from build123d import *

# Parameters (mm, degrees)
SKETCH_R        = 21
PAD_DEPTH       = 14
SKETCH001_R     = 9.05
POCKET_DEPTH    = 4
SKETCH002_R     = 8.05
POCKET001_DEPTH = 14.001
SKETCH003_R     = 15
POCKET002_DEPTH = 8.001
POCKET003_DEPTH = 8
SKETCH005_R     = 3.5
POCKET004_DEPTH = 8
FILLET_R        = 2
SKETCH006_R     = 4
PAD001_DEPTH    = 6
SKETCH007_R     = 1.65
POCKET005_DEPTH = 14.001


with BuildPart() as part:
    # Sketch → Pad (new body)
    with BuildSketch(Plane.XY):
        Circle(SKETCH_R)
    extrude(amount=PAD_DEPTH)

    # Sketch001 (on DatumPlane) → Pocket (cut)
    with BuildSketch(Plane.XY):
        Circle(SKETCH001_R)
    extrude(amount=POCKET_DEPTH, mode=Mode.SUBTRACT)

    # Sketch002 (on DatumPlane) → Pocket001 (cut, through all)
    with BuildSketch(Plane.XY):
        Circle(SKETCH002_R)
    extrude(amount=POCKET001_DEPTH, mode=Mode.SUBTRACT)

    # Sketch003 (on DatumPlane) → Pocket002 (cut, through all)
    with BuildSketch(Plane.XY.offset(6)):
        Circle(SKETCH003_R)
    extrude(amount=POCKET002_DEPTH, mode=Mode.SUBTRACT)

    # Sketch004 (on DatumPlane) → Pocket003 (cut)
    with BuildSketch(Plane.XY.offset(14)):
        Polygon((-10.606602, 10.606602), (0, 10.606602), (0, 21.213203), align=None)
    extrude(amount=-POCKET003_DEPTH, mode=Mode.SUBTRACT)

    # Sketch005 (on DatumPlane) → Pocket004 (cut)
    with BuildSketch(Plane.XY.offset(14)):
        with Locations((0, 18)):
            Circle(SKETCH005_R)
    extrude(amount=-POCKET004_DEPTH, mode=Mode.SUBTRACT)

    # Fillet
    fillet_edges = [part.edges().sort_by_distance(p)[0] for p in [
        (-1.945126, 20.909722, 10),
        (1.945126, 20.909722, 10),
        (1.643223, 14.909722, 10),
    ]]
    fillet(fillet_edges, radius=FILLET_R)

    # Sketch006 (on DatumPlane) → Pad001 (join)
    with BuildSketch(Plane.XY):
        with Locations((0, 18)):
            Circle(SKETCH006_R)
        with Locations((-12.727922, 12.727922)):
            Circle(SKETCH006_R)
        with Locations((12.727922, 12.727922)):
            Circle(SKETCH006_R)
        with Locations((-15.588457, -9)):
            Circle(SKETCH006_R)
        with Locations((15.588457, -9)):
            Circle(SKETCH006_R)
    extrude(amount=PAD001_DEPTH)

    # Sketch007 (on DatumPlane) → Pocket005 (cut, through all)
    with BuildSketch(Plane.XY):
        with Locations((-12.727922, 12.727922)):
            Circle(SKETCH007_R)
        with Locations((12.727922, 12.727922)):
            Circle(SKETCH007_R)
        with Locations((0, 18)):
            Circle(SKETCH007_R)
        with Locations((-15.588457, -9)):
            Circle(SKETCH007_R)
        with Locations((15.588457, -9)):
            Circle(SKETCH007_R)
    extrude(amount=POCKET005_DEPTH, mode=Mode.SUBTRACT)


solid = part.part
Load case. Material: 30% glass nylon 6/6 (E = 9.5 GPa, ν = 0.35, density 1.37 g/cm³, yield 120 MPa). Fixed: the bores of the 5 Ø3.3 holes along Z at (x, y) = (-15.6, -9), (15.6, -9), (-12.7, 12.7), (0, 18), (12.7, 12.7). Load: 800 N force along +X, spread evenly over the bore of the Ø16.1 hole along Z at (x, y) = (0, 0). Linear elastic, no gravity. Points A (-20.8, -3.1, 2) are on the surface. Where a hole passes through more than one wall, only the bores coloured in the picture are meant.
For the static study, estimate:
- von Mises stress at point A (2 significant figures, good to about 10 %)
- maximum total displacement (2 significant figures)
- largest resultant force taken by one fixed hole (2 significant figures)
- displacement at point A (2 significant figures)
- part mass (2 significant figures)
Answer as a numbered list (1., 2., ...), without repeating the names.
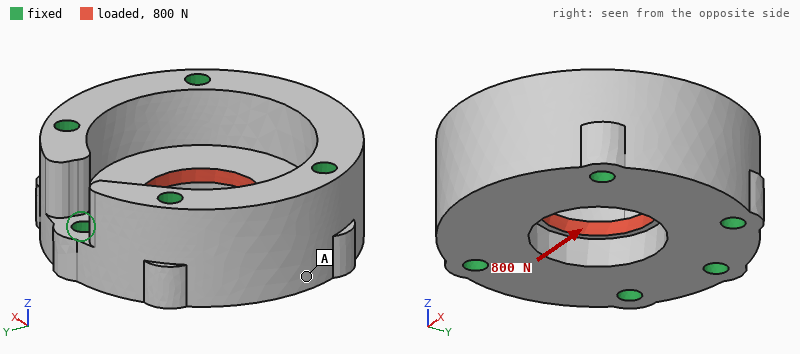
1. 1.5 MPa
2. 8.6 µm
3. 220 N
4. 2.1 µm
5. 16 g
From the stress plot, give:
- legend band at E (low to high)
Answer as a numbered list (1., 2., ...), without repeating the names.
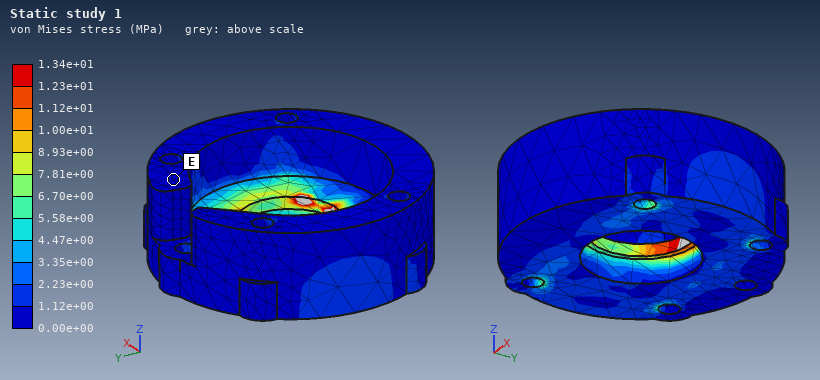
1. 0.00e+00 to 1.12e+00 MPa
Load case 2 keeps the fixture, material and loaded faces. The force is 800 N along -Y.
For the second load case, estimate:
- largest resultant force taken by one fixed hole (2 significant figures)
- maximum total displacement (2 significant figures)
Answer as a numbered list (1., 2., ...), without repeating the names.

1. 200 N
2. 11 µm
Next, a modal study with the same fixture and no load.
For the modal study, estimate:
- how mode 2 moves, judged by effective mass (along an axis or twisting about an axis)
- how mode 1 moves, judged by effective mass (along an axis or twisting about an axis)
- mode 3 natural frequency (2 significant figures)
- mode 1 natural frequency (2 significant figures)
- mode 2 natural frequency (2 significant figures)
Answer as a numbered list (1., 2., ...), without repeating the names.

1. along Y
2. along Z
3. 24 kHz
4. 15 kHz
5. 22 kHz
